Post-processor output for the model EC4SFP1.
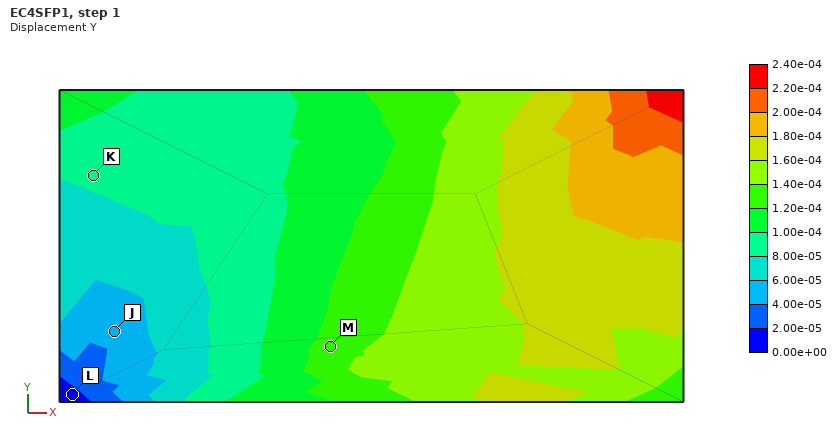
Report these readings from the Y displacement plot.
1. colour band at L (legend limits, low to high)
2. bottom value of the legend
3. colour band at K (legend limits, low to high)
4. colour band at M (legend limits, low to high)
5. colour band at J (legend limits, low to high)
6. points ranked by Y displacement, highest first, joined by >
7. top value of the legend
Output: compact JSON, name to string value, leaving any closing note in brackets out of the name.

{"colour band at L": "0.00e+00 to 2.00e-05", "bottom value of the legend": "0.00e+00", "colour band at K": "8.00e-05 to 1.00e-04", "colour band at M": "1.20e-04 to 1.40e-04", "colour band at J": "4.00e-05 to 6.00e-05", "points ranked by Y displacement, highest first, joined by >": "M > K > J > L", "top value of the legend": "2.40e-04"}
